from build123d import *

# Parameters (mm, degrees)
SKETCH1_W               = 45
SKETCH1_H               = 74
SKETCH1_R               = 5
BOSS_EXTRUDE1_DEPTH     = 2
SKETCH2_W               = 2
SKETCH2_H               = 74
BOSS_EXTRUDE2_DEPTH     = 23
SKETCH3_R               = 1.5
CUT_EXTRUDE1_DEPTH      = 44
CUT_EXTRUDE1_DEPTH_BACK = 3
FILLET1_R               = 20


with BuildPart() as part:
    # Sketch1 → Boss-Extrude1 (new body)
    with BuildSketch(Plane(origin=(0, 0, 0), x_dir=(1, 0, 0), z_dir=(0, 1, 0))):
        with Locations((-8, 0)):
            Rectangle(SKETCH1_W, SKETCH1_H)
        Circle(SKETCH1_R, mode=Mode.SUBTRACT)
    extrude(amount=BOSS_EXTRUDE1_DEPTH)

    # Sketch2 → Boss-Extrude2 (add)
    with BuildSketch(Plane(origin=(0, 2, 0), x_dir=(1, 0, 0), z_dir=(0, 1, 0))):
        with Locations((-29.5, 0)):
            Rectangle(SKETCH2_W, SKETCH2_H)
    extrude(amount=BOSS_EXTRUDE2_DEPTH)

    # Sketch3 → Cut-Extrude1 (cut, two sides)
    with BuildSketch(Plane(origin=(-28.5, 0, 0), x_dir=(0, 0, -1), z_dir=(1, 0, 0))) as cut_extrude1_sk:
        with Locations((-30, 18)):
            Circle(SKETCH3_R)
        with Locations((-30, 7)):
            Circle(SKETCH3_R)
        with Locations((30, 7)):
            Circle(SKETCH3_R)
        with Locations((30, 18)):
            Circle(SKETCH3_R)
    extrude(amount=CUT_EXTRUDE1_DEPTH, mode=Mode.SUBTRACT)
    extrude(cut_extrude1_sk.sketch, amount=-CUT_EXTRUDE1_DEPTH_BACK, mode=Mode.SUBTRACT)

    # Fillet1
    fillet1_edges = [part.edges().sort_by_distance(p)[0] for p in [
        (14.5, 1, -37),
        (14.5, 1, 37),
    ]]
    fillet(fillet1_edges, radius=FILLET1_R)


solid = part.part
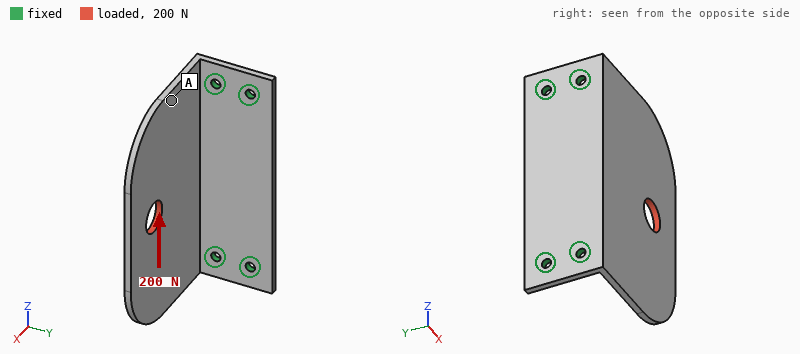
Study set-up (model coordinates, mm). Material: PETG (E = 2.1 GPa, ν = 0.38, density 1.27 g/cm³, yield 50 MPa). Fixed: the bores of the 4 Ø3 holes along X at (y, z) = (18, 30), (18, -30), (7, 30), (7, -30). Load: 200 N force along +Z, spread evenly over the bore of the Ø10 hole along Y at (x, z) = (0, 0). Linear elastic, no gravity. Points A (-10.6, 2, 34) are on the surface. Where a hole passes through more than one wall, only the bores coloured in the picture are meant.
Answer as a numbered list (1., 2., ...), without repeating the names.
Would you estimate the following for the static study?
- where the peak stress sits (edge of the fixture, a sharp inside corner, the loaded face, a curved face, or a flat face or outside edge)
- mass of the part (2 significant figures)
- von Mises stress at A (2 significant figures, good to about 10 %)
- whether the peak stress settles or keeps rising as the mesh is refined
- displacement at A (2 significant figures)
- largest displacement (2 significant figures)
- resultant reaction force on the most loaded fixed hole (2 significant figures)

1. edge of the fixture
2. 12 g
3. 3.5 MPa
4. keeps rising
5. 0.75 mm
6. 1.0 mm
7. 130 N
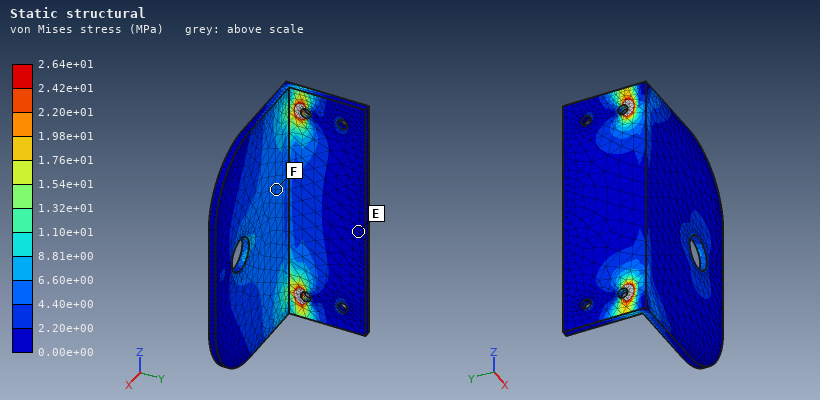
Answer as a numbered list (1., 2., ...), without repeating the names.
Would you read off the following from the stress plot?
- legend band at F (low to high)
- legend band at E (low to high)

1. 4.40e+00 to 6.60e+00 MPa
2. 0.00e+00 to 2.20e+00 MPa
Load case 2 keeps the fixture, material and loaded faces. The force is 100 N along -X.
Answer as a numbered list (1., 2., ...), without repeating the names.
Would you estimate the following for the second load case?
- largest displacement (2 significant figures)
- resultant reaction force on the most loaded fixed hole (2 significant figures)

1. 1.0 mm
2. 62 N
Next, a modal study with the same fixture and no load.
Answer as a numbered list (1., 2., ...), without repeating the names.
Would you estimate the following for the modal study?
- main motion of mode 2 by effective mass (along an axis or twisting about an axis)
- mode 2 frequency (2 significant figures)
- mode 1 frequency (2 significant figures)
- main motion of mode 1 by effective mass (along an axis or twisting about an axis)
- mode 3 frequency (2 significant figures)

1. twisting about X
2. 380 Hz
3. 190 Hz
4. along Y
5. 830 Hz
